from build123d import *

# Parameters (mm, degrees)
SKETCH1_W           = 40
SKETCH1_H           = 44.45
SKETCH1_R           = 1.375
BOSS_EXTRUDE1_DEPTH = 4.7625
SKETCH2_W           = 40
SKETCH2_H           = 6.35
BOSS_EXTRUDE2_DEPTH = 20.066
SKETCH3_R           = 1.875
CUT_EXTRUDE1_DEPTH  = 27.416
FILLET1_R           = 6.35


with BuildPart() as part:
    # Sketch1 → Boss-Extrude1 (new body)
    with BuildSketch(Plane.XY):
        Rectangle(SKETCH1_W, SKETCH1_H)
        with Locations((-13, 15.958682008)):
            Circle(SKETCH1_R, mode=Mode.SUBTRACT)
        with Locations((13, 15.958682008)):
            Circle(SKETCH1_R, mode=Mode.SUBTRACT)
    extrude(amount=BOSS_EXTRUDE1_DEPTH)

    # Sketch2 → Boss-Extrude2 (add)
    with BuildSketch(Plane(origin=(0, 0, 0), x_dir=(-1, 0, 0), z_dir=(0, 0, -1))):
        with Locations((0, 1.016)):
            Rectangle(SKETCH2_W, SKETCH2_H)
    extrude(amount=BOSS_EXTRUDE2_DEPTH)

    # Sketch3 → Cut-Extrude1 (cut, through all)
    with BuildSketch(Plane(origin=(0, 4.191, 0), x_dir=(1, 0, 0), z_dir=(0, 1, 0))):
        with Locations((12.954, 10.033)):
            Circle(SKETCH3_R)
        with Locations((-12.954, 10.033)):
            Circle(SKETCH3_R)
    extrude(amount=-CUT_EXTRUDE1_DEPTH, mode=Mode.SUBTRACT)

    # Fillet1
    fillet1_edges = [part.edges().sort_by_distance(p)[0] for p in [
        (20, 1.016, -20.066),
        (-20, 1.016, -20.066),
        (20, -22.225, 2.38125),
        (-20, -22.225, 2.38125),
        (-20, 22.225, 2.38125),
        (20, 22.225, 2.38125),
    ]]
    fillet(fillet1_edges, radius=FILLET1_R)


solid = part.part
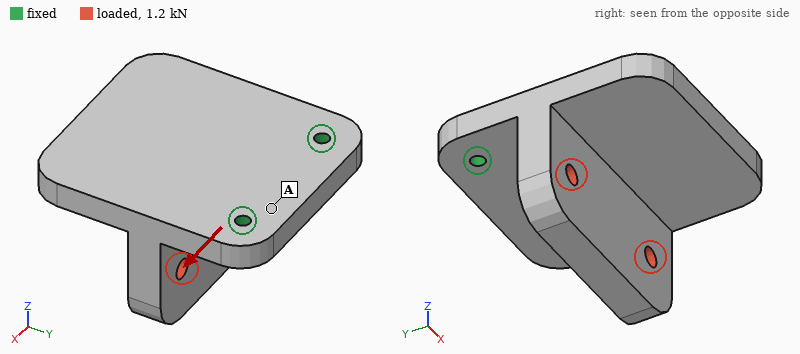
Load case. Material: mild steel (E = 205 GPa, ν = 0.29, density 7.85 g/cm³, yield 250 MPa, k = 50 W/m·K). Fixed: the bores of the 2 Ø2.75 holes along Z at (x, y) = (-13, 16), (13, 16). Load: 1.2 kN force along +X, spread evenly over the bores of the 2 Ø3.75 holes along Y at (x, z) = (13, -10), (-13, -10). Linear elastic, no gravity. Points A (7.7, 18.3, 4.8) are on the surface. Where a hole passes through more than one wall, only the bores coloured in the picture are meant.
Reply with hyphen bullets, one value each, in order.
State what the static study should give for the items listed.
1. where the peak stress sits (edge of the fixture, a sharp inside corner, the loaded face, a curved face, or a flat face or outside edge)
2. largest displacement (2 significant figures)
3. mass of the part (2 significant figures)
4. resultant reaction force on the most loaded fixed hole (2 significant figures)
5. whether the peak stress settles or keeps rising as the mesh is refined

- edge of the fixture
- 17 µm
- 100 g
- 1.0 kN
- keeps rising
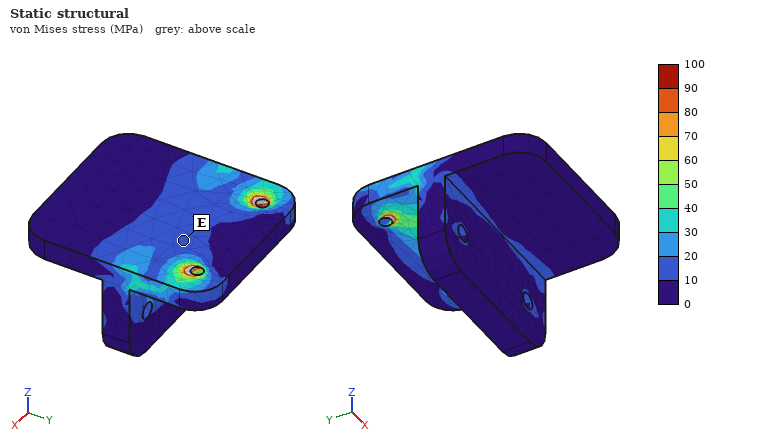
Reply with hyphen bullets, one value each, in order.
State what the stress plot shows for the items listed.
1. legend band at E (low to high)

- 10 to 20 MPa
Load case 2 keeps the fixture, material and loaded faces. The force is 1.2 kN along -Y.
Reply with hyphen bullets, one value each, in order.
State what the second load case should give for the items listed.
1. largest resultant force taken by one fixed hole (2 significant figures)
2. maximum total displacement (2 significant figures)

- 600 N
- 0.10 mm
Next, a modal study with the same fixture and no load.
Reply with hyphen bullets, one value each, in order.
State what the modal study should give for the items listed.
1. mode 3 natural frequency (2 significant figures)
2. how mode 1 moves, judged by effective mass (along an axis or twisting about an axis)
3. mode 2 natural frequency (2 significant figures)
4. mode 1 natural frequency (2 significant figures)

- 9400 Hz
- along Z
- 5600 Hz
- 2100 Hz
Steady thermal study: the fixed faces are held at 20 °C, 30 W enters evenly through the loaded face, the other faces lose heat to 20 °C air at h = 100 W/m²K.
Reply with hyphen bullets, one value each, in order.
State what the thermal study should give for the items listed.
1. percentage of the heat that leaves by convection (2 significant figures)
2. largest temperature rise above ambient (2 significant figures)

- 52 %
- 55 K
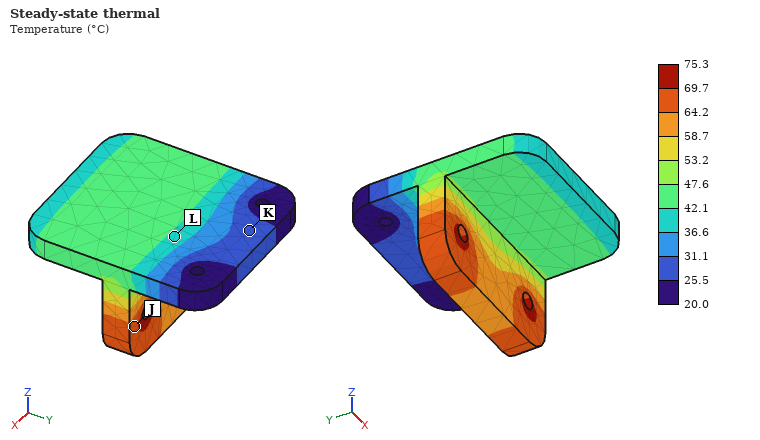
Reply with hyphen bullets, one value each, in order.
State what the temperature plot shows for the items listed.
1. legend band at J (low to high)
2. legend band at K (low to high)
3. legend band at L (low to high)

- 64.2 to 69.7 °C
- 25.5 to 31.1 °C
- 36.6 to 42.1 °C
